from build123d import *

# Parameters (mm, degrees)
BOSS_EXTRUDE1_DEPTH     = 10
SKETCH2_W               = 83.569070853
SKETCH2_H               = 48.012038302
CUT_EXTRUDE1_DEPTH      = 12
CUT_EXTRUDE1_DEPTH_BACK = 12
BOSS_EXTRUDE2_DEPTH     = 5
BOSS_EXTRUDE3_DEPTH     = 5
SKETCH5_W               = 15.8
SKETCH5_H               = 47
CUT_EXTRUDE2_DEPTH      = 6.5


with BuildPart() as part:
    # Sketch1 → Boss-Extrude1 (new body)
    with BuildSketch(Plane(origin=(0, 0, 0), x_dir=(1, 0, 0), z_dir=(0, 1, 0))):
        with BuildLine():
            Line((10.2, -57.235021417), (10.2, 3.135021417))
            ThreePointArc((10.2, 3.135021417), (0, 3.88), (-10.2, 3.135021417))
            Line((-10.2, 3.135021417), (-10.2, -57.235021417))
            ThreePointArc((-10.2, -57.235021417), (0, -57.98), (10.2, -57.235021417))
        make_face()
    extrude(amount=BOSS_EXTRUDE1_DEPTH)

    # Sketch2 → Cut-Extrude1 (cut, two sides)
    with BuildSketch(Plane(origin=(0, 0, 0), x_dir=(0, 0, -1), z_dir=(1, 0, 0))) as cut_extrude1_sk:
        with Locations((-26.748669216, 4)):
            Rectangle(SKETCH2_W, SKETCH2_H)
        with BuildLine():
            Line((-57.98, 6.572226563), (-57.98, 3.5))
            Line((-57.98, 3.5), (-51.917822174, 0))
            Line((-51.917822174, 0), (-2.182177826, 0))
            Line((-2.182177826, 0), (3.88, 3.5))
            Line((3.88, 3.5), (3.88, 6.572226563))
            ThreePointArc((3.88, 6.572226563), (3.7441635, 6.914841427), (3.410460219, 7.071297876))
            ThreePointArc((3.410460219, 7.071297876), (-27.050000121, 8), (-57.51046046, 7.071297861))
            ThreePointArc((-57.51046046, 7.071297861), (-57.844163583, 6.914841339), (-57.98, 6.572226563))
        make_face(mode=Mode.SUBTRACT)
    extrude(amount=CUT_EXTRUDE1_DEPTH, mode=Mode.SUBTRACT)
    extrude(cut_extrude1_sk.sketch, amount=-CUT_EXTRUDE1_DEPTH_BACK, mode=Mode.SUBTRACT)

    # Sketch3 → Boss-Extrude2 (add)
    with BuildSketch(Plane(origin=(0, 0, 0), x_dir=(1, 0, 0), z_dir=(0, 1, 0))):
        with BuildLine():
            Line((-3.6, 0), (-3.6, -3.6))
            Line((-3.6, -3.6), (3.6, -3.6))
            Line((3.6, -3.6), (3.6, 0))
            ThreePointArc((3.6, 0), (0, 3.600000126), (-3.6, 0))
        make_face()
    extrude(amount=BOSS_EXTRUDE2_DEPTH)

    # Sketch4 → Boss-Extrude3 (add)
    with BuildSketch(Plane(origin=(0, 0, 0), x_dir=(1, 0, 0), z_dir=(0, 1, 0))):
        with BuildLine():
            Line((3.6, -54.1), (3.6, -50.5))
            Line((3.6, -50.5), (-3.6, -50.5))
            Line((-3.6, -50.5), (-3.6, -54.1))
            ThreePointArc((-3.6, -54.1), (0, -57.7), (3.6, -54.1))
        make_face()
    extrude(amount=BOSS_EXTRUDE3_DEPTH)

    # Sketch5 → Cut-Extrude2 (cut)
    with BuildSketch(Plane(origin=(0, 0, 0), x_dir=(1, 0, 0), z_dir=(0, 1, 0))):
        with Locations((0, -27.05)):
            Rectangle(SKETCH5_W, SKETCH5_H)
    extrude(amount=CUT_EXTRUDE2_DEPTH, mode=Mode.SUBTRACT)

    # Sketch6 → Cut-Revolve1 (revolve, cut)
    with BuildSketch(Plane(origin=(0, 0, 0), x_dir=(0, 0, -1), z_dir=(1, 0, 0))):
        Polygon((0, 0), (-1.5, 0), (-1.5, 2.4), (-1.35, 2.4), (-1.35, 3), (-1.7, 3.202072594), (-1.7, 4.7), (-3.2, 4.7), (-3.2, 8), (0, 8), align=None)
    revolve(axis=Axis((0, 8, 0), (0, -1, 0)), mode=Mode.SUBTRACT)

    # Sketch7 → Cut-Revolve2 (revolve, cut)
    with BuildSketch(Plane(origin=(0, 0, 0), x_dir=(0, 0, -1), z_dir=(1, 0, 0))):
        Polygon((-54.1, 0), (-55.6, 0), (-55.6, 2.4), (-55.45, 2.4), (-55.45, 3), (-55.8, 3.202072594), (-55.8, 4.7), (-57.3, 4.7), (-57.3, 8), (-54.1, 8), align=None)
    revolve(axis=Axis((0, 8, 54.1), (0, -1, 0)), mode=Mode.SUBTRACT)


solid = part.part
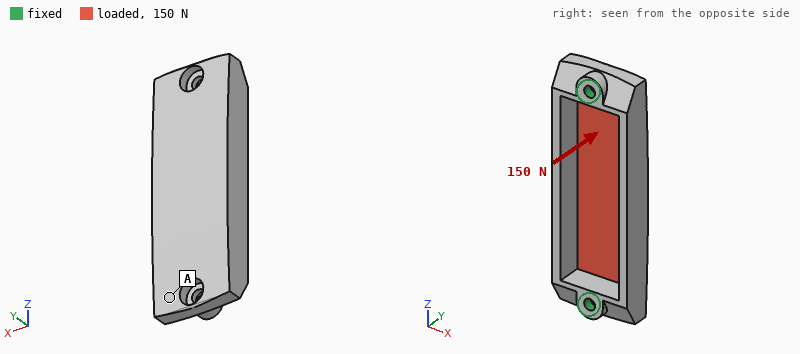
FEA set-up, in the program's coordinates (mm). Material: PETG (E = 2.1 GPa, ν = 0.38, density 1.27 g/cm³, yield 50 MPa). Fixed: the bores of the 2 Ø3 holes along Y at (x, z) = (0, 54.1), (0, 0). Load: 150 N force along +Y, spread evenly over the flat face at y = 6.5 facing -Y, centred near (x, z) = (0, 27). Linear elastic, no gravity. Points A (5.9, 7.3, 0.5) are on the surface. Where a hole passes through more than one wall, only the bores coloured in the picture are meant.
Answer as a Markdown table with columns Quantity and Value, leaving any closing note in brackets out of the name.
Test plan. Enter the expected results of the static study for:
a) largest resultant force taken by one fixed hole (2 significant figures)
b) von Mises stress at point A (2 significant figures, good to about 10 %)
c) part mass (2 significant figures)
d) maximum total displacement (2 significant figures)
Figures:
| Quantity | Value |
|---|---|
| largest resultant force taken by one fixed hole | 90 N |
| von Mises stress at point A | 4.1 MPa |
| part mass | 5.4 g |
| maximum total displacement | 0.53 mm |
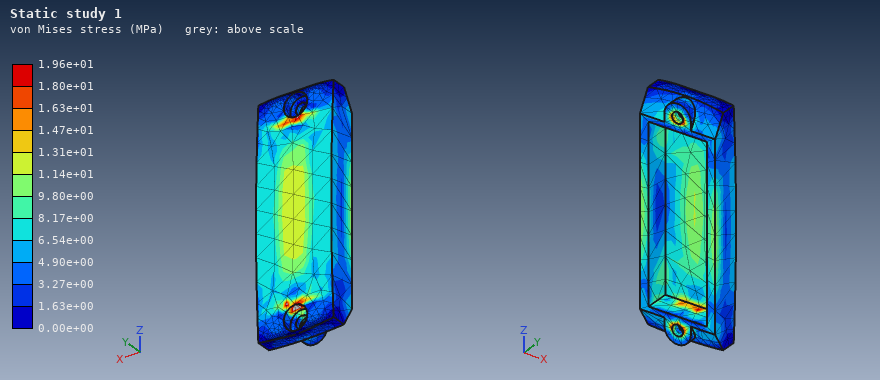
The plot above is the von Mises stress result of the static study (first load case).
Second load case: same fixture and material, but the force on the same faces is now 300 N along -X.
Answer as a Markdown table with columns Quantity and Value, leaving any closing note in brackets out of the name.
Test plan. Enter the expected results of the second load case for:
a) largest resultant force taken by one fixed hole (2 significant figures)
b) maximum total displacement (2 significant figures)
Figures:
| Quantity | Value |
|---|---|
| largest resultant force taken by one fixed hole | 150 N |
| maximum total displacement | 0.38 mm |
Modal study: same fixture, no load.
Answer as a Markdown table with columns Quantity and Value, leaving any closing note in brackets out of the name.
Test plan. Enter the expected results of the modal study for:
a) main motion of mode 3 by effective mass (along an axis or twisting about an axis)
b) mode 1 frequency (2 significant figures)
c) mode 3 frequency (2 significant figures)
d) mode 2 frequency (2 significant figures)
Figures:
| Quantity | Value |
|---|---|
| main motion of mode 3 by effective mass | along X |
| mode 1 frequency | 1900 Hz |
| mode 3 frequency | 2600 Hz |
| mode 2 frequency | 1900 Hz |
